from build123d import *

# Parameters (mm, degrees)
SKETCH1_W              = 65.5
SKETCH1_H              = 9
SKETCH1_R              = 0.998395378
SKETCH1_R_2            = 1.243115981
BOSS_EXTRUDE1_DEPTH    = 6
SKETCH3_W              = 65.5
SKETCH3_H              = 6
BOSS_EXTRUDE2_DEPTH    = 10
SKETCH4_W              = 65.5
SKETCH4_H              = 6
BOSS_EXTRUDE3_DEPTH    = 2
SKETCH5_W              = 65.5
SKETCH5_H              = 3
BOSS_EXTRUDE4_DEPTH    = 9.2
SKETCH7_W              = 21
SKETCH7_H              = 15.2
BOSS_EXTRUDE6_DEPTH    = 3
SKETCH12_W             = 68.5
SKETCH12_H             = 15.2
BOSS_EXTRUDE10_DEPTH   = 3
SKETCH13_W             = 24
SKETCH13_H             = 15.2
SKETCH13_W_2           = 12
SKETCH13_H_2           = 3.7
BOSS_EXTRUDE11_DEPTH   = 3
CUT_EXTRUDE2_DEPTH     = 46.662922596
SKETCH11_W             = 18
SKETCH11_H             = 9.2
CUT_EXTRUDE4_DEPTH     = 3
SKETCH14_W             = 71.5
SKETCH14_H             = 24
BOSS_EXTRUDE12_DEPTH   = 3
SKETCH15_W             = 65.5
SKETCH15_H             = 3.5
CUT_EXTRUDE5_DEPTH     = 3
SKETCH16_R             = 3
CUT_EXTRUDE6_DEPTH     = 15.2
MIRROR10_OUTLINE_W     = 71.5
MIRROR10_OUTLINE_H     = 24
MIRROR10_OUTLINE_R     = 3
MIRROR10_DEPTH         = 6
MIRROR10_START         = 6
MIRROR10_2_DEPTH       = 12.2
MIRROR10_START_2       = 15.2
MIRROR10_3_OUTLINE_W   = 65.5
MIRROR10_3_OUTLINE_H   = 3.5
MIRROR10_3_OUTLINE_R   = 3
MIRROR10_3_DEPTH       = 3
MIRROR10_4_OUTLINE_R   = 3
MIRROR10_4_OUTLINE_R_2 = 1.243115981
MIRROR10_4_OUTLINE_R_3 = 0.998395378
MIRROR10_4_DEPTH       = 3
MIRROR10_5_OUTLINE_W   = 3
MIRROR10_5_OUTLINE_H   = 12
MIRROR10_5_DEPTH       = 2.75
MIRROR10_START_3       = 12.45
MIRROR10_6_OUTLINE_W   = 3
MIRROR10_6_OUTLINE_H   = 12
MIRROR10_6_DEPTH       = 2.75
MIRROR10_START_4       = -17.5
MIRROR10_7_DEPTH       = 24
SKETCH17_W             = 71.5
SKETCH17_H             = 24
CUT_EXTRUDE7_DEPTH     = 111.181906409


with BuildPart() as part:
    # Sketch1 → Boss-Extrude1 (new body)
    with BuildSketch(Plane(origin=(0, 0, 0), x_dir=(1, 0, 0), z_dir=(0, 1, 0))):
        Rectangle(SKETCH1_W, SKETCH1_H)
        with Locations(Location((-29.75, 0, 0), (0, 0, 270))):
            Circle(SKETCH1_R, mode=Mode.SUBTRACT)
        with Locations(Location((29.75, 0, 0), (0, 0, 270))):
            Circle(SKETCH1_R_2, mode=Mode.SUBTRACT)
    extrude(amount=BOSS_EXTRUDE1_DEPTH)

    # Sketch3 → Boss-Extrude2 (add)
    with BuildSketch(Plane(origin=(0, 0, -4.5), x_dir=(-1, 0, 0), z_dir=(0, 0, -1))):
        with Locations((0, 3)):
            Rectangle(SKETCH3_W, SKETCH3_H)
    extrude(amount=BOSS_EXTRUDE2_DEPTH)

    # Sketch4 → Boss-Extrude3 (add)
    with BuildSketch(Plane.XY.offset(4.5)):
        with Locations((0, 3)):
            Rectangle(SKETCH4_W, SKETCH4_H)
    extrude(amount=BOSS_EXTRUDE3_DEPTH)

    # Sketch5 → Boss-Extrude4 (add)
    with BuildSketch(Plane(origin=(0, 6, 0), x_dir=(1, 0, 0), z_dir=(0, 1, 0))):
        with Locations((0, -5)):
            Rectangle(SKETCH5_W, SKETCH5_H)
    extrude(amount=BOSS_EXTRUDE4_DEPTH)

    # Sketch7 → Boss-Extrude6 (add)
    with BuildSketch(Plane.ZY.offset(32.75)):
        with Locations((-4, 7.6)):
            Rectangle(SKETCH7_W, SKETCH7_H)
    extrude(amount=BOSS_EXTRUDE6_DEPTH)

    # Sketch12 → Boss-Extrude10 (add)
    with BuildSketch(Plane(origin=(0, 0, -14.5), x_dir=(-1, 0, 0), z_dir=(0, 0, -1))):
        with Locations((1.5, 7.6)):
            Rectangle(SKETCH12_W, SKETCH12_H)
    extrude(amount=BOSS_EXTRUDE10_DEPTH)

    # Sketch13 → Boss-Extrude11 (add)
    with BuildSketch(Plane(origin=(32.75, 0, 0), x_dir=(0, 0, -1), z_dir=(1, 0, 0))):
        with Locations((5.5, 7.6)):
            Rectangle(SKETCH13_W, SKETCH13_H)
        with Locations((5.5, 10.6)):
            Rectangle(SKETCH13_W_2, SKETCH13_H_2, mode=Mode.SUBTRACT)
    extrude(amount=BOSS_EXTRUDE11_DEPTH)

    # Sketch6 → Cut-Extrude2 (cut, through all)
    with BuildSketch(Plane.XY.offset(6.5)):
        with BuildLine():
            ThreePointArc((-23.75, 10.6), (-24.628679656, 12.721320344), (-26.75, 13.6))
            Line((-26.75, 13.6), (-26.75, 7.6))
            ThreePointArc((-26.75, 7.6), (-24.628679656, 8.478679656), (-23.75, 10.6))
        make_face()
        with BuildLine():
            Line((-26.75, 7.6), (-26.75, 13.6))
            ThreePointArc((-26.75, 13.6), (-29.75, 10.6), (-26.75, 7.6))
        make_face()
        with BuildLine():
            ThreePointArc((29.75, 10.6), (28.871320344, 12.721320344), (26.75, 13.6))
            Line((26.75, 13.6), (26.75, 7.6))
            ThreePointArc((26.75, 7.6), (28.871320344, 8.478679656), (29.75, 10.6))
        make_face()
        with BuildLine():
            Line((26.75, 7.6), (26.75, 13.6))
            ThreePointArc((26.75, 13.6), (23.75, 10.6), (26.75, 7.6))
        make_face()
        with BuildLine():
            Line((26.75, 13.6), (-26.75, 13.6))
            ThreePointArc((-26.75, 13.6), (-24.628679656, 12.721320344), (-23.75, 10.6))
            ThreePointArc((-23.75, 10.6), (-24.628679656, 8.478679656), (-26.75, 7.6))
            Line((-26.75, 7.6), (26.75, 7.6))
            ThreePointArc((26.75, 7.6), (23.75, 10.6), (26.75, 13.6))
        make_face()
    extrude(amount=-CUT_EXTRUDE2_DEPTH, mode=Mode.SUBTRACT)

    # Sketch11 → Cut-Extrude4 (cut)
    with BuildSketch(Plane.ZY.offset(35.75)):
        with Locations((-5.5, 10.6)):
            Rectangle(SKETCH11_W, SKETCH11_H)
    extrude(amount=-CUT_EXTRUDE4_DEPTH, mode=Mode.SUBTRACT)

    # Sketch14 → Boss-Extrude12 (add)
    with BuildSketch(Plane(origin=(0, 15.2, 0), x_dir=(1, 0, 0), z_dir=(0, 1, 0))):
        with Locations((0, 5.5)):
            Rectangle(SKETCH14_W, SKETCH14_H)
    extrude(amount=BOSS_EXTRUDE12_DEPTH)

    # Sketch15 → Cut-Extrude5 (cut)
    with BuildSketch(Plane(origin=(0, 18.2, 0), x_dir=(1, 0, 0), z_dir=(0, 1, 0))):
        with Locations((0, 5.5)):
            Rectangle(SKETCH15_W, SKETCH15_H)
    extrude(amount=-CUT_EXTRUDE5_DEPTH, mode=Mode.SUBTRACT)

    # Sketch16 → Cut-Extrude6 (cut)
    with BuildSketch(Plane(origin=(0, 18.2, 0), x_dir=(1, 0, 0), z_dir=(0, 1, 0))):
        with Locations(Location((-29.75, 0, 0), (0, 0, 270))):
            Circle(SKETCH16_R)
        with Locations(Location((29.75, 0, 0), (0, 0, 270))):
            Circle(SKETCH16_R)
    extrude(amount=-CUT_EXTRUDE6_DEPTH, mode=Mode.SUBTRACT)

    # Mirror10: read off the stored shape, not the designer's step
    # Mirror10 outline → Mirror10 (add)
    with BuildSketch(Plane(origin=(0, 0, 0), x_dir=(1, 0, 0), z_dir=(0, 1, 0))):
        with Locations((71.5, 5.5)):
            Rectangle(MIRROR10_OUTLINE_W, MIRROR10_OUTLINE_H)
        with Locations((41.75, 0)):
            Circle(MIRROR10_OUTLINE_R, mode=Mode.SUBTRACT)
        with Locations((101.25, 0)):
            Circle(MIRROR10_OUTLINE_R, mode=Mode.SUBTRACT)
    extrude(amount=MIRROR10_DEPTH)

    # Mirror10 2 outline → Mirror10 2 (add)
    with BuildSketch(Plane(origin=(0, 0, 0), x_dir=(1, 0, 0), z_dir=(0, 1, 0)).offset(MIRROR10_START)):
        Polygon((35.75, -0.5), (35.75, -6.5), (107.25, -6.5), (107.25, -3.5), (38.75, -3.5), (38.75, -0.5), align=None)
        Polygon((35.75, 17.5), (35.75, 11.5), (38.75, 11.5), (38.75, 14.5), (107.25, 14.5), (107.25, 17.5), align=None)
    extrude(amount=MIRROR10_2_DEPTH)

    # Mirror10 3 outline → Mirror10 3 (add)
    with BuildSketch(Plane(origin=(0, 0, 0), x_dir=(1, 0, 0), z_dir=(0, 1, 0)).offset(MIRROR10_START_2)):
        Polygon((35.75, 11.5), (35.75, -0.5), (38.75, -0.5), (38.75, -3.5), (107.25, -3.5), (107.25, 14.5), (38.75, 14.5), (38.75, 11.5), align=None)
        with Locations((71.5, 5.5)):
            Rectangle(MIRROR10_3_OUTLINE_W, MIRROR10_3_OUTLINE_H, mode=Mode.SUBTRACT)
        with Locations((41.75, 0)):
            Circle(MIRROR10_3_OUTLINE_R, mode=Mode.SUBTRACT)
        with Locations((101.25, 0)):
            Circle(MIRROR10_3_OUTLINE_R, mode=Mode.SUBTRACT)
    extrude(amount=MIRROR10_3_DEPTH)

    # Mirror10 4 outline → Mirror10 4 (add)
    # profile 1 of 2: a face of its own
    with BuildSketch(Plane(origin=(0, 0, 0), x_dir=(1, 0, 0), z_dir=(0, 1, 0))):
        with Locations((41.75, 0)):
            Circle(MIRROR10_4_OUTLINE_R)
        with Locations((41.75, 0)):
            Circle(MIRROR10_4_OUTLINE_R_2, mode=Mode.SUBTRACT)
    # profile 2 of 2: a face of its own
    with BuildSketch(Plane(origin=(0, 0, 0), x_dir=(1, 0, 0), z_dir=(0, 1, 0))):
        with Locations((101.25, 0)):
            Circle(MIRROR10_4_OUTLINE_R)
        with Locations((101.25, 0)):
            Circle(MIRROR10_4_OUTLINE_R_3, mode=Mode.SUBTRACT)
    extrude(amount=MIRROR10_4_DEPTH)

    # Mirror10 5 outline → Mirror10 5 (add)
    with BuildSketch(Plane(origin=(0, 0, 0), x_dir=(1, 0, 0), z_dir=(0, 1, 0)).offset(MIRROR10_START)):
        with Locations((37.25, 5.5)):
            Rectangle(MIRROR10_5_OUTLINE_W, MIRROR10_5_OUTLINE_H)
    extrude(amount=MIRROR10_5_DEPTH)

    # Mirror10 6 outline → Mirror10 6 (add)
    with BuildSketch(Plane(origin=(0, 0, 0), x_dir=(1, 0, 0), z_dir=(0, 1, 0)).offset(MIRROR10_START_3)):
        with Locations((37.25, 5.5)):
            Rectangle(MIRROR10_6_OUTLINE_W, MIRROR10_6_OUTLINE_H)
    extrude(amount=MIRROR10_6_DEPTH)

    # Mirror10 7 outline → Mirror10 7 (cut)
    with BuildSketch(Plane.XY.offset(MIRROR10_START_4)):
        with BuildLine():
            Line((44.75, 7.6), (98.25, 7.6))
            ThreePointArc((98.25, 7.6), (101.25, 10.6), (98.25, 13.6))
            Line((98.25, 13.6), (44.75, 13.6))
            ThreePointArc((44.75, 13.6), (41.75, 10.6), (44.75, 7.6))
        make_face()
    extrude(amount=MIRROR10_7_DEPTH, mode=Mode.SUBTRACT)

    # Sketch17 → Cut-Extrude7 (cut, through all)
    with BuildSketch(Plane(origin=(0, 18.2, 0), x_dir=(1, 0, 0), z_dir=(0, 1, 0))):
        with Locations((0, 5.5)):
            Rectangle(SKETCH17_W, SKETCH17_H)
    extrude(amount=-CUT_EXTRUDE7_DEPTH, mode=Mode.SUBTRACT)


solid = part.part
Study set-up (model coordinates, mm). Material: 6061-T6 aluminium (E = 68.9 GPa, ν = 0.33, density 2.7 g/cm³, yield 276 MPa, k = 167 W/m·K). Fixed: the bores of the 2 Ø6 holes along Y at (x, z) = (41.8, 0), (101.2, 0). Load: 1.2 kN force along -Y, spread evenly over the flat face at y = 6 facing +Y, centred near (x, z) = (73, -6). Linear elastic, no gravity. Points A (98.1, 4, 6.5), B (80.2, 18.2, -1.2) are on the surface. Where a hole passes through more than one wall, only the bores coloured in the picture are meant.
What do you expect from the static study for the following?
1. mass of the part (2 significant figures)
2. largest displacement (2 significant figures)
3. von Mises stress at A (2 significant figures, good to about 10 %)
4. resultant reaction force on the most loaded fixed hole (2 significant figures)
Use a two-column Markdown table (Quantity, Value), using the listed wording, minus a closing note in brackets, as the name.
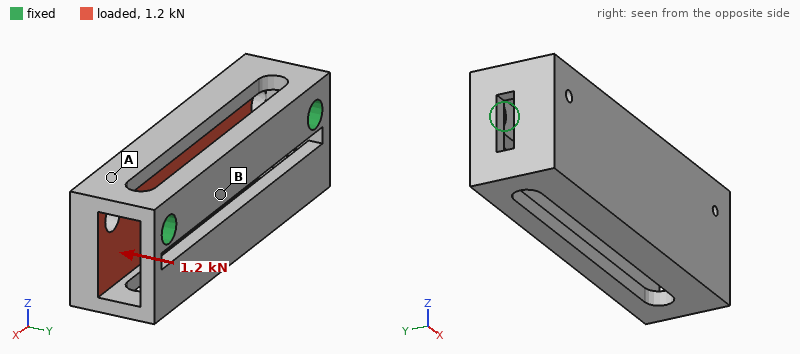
| Quantity | Value |
|---|---|
| mass of the part | 45 g |
| largest displacement | 0.20 mm |
| von Mises stress at A | 40 MPa |
| resultant reaction force on the most loaded fixed hole | 670 N |
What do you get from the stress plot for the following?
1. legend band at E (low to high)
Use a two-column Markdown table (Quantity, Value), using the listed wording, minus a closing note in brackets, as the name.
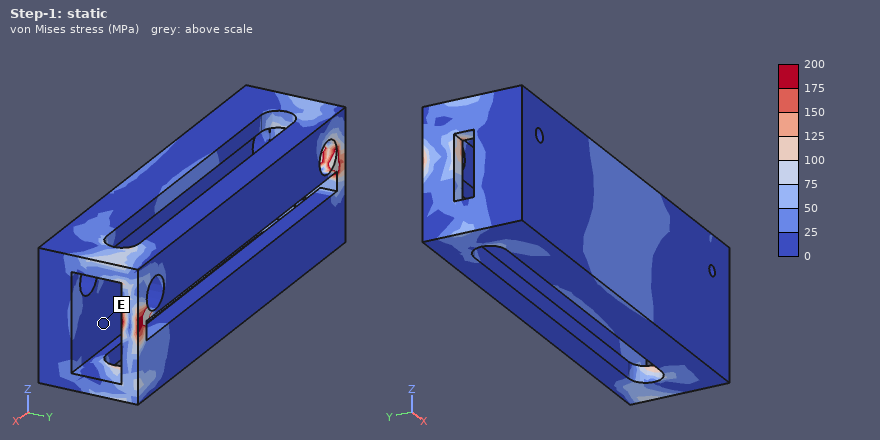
| Quantity | Value |
|---|---|
| legend band at E | 0 to 25 MPa |
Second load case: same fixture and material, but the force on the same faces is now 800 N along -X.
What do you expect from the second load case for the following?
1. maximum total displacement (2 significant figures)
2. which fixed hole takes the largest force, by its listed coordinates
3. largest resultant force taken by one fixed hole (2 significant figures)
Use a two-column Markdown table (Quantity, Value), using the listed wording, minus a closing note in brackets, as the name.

| Quantity | Value |
|---|---|
| maximum total displacement | 30 µm |
| which fixed hole takes the largest force, by its listed coordinates | (41.8, 0) |
| largest resultant force taken by one fixed hole | 450 N |
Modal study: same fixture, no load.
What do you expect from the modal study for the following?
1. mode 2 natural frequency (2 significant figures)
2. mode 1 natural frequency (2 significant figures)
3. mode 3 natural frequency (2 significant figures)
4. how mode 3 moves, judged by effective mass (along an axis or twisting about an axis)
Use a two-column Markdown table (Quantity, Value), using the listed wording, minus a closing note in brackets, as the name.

| Quantity | Value |
|---|---|
| mode 2 natural frequency | 4100 Hz |
| mode 1 natural frequency | 2000 Hz |
| mode 3 natural frequency | 4600 Hz |
| how mode 3 moves, judged by effective mass | along X |
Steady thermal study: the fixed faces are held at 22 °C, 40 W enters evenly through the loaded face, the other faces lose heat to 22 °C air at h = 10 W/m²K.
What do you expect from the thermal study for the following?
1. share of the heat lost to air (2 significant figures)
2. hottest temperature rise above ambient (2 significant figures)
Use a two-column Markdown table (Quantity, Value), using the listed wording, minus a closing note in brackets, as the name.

| Quantity | Value |
|---|---|
| share of the heat lost to air | 6.8 % |
| hottest temperature rise above ambient | 55 K |
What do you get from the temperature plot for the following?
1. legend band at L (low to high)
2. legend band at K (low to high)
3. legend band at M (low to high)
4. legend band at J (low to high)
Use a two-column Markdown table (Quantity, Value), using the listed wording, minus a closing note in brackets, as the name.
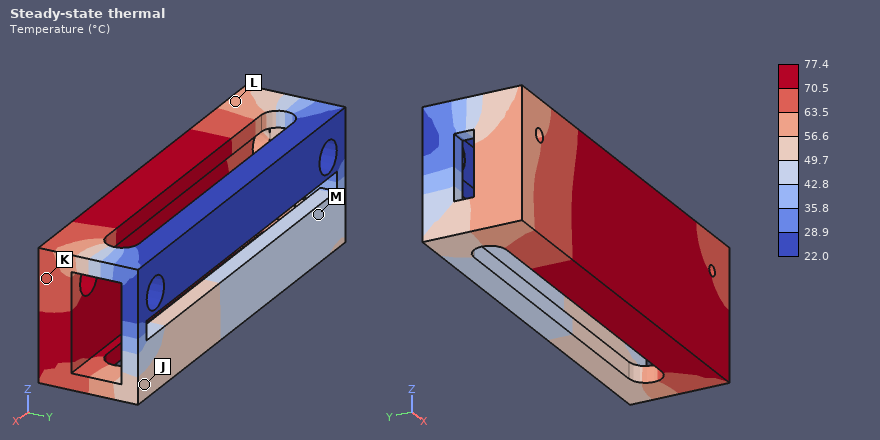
| Quantity | Value |
|---|---|
| legend band at L | 56.6 to 63.5 °C |
| legend band at K | 63.5 to 70.5 °C |
| legend band at M | 42.8 to 49.7 °C |
| legend band at J | 49.7 to 56.6 °C |
